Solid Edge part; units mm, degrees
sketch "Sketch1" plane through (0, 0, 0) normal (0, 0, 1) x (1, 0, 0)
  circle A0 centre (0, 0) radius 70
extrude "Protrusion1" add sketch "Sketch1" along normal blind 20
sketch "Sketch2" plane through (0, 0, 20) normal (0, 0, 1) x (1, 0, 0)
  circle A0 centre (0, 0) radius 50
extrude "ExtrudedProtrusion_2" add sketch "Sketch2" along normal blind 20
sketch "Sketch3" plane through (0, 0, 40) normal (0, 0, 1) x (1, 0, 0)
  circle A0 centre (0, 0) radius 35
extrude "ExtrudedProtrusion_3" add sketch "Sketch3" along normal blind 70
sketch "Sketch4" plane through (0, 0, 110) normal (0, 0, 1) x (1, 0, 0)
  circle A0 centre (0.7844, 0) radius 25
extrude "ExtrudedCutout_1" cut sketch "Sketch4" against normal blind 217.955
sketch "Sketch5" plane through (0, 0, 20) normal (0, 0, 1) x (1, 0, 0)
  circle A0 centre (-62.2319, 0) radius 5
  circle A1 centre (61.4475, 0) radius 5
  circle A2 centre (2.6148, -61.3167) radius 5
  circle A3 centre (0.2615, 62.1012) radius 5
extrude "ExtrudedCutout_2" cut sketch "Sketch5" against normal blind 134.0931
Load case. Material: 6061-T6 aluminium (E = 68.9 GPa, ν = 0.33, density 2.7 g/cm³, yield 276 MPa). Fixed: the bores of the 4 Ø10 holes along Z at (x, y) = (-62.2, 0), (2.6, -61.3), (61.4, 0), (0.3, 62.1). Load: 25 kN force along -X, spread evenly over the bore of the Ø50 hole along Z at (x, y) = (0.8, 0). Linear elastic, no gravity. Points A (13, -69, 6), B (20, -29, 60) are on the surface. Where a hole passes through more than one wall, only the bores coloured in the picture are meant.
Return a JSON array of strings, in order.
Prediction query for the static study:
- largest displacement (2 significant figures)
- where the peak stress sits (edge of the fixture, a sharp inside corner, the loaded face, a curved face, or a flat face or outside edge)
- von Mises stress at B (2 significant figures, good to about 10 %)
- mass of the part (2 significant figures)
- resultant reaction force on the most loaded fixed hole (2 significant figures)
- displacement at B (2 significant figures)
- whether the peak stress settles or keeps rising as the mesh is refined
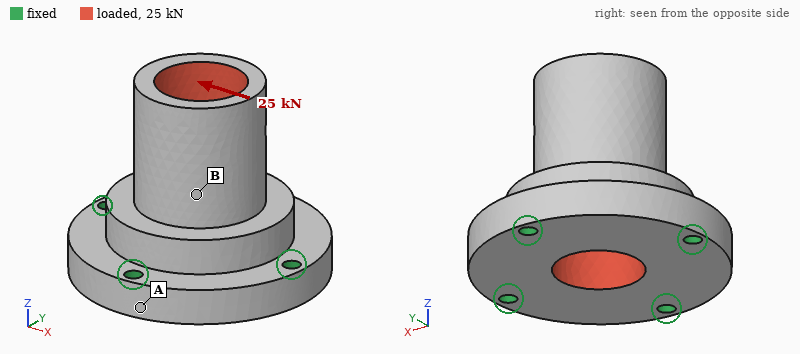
["75 µm", "edge of the fixture", "14 MPa", "1.4 kg", "13 kN", "34 µm", "keeps rising"]
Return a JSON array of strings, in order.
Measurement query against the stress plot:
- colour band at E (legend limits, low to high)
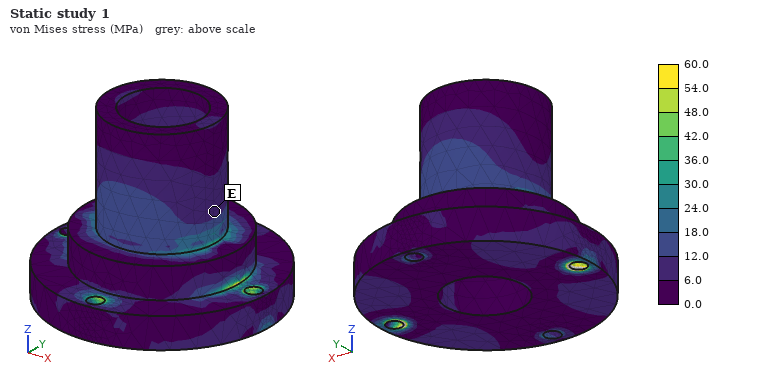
["6.0 to 12.0 MPa"]
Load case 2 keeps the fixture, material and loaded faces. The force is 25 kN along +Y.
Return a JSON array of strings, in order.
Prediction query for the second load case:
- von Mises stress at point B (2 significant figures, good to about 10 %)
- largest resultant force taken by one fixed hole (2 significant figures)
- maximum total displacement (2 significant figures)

["12 MPa", "13 kN", "75 µm"]
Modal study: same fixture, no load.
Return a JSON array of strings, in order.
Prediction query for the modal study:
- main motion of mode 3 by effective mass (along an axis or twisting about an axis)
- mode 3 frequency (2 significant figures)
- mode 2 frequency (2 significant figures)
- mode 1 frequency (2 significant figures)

["along Z", "7000 Hz", "4500 Hz", "4400 Hz"]
